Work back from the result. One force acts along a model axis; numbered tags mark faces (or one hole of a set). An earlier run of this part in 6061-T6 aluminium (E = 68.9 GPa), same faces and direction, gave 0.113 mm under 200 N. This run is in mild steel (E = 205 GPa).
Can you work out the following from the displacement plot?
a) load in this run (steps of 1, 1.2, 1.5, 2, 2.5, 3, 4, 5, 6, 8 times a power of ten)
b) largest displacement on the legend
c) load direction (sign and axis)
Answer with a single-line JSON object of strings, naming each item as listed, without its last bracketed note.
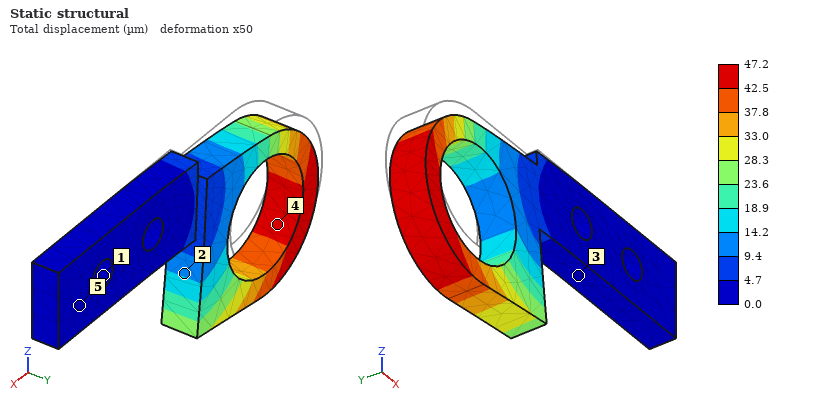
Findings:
{"load in this run": "250 N", "largest displacement on the legend": "47.2 µm", "load direction": "-Z"}
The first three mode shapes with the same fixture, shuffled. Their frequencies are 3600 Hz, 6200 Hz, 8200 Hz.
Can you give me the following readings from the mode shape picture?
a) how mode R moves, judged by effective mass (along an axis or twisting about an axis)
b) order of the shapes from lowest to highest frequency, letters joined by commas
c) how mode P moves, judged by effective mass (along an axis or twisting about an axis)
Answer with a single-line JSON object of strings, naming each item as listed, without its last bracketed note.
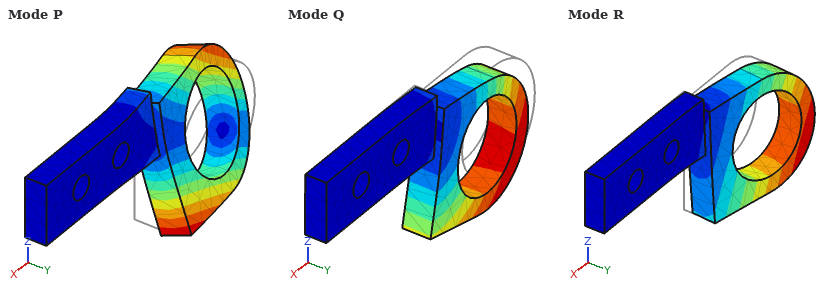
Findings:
{"how mode R moves, judged by effective mass": "along Y", "order of the shapes from lowest to highest frequency, letters joined by commas": "R, Q, P", "how mode P moves, judged by effective mass": "twisting about X"}
